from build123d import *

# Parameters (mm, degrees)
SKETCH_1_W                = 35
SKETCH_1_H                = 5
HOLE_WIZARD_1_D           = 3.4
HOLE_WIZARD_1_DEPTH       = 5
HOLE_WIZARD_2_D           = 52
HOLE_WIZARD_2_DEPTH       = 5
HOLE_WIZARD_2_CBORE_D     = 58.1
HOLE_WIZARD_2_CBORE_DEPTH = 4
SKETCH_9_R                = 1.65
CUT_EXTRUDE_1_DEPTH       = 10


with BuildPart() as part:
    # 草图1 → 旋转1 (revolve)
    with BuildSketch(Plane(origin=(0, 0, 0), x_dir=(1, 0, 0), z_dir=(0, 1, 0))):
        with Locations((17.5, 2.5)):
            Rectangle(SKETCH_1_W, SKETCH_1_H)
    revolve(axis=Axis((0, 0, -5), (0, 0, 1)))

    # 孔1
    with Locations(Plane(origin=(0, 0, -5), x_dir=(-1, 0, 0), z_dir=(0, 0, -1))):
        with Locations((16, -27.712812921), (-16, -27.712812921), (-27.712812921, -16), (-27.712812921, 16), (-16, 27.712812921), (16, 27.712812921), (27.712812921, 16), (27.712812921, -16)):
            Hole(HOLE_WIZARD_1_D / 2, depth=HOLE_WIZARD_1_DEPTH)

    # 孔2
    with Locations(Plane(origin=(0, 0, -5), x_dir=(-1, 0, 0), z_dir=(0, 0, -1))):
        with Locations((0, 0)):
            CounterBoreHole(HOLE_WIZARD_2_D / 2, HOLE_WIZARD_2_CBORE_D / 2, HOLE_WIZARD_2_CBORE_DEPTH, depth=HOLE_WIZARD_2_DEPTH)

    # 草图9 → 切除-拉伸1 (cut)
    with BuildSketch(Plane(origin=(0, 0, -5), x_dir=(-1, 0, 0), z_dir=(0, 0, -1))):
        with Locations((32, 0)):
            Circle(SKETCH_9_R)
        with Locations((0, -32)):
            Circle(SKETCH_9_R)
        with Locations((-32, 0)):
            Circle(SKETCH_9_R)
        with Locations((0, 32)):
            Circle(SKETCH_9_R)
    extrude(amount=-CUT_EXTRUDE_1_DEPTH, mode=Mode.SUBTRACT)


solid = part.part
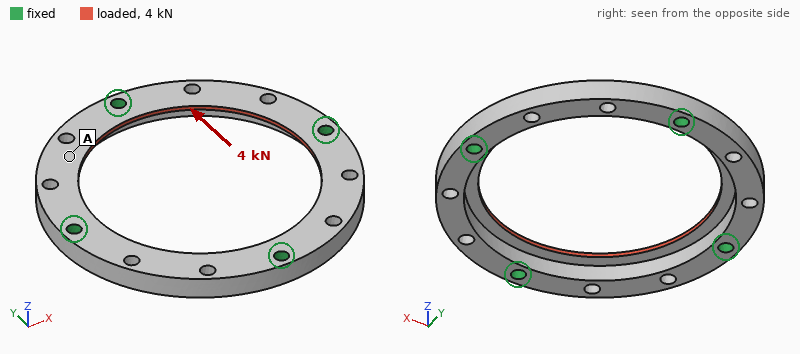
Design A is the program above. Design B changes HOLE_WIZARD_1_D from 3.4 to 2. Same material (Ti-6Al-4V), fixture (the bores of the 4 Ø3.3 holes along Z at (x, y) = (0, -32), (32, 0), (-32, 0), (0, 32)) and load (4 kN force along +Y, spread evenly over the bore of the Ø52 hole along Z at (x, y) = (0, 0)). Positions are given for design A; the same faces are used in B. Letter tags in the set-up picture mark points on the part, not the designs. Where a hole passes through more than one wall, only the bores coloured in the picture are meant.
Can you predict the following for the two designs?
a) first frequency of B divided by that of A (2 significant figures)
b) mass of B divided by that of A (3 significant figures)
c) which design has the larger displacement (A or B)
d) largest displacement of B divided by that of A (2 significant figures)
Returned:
1.00
1.04
A
0.91
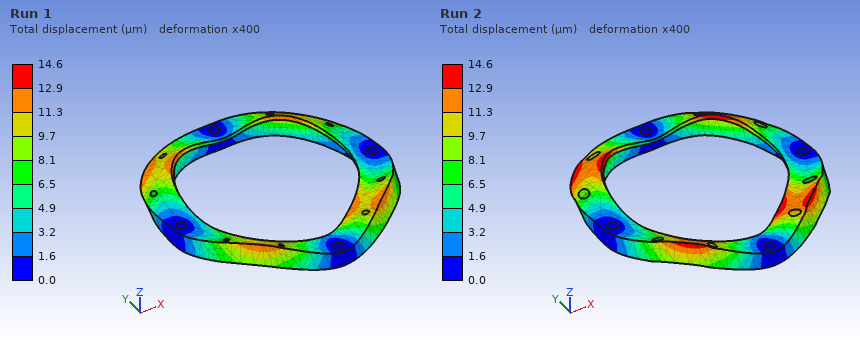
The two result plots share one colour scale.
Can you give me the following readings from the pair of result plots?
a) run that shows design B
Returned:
Run 1
